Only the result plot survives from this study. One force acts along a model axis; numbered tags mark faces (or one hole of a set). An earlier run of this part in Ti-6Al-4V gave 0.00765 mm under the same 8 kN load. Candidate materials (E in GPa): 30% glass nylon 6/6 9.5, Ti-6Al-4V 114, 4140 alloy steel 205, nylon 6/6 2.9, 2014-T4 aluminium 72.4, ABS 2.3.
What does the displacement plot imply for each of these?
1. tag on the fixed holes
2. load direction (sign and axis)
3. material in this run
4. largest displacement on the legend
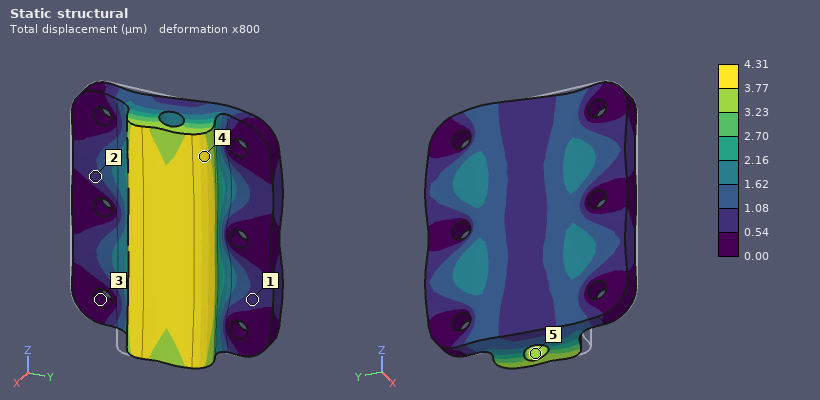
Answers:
3
+Y
4140 alloy steel
4.31 µm
